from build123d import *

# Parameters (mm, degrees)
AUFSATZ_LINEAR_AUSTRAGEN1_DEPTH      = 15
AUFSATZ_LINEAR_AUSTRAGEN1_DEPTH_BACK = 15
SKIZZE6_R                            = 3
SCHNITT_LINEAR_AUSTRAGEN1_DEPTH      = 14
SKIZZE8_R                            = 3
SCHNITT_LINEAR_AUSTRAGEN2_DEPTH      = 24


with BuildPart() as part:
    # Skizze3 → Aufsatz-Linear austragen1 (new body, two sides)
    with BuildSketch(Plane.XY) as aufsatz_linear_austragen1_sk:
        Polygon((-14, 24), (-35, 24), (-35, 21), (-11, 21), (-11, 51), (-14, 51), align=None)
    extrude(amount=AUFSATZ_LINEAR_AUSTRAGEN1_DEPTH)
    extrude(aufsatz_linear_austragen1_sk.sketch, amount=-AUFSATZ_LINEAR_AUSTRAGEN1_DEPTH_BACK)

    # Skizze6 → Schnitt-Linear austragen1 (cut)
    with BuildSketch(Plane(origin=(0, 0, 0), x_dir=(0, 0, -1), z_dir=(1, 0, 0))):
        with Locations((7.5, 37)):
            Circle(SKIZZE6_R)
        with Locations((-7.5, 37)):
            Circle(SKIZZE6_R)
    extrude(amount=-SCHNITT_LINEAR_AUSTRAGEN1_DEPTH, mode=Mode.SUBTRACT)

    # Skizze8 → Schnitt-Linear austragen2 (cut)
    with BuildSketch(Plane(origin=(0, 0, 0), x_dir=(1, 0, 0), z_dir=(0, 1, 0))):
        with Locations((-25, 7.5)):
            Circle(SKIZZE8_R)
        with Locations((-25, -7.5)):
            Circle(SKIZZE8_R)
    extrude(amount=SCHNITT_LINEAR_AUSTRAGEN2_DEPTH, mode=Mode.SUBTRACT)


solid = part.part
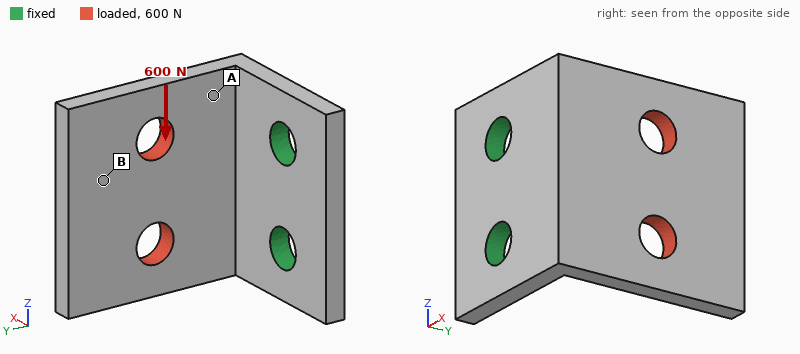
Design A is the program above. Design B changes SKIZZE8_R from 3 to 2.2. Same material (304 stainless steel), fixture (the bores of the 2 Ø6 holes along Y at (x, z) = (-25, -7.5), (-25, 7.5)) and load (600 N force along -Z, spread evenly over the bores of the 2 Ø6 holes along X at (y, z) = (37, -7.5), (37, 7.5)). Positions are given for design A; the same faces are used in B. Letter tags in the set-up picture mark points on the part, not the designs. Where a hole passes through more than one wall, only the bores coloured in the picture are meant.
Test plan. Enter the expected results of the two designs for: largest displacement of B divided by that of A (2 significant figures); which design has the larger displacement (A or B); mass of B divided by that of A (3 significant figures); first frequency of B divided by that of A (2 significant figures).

1.2
B
1.02
0.96
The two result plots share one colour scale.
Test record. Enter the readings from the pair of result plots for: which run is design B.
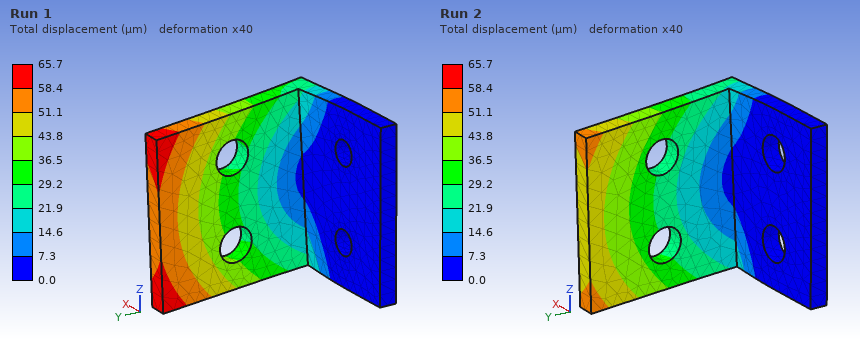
Run 1
